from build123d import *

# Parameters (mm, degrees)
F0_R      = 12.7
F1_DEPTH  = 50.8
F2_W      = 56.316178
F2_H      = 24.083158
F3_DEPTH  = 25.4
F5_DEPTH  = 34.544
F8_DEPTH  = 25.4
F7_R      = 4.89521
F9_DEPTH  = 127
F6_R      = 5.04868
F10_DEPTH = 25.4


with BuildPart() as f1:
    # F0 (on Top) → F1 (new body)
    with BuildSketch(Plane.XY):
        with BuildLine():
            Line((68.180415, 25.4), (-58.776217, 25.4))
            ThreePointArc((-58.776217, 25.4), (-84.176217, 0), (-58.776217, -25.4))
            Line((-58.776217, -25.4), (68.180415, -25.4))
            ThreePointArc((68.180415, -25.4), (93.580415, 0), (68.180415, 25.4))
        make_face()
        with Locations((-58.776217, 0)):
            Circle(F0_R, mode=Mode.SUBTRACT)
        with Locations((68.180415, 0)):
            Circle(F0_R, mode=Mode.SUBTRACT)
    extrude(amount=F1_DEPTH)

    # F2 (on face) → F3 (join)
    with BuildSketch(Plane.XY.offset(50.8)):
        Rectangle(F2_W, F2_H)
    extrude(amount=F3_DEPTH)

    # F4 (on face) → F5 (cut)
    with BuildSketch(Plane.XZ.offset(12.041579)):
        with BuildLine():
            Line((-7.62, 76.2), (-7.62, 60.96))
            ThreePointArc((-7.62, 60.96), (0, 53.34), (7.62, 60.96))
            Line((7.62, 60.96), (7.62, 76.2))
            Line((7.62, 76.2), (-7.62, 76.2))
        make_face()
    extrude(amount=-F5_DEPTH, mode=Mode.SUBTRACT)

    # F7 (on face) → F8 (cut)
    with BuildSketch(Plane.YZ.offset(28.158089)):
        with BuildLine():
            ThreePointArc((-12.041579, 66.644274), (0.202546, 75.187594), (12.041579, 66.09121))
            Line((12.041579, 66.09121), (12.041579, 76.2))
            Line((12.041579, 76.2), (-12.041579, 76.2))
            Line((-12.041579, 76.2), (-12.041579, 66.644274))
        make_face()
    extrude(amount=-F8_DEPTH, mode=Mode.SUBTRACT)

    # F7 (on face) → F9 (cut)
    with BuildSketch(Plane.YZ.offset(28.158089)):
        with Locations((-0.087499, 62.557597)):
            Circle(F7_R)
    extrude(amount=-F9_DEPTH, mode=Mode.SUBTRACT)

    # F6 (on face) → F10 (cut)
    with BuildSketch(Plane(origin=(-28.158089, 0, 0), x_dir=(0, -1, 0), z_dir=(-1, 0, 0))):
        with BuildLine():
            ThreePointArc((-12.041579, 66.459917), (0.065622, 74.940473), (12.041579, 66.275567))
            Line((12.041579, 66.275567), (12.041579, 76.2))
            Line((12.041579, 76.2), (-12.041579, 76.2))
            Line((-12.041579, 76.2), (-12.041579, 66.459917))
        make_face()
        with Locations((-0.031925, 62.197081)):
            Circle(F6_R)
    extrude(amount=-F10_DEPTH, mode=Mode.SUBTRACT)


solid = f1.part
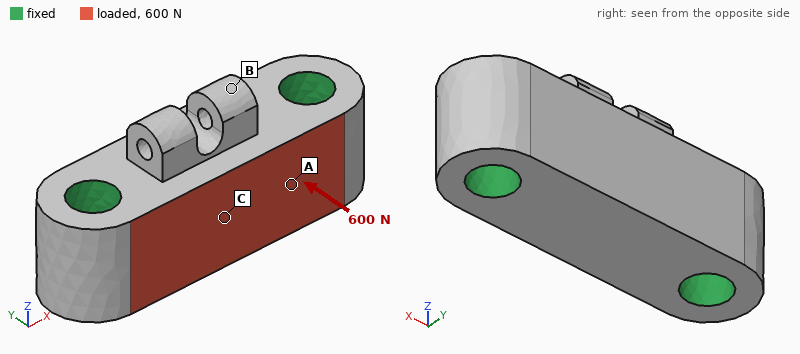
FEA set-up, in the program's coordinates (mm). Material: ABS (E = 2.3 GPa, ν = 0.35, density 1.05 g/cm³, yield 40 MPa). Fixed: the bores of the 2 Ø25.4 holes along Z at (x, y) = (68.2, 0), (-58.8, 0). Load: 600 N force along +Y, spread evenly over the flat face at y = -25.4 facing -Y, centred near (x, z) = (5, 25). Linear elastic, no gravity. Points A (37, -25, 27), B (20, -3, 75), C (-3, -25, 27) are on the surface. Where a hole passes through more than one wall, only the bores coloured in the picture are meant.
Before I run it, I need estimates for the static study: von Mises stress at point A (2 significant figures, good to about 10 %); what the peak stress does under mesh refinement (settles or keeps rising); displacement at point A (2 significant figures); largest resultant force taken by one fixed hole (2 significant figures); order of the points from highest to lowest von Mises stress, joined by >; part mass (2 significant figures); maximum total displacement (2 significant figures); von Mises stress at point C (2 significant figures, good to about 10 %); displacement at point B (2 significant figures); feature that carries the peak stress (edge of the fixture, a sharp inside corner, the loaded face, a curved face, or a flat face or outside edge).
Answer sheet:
0.092 MPa
keeps rising
4.7 µm
300 N
C > A > B
420 g
7.1 µm
0.17 MPa
6.5 µm
edge of the fixture
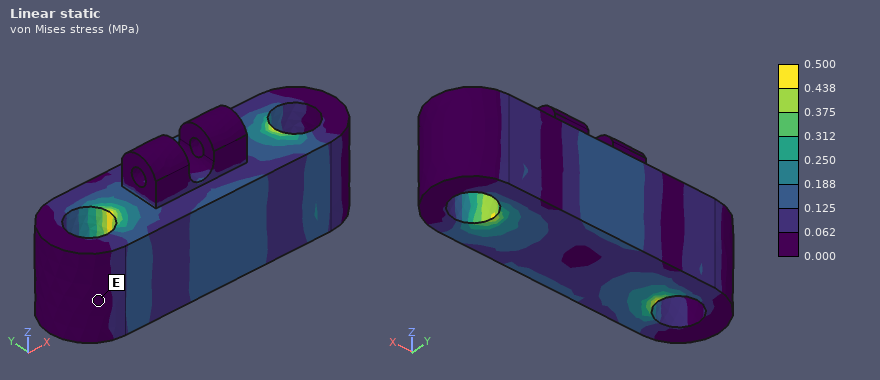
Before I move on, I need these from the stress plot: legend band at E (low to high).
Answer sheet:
0.000 to 0.062 MPa
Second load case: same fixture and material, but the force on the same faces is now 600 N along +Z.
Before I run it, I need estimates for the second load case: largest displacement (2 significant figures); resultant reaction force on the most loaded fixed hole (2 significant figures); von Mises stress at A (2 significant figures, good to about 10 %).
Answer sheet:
15 µm
300 N
0.41 MPa
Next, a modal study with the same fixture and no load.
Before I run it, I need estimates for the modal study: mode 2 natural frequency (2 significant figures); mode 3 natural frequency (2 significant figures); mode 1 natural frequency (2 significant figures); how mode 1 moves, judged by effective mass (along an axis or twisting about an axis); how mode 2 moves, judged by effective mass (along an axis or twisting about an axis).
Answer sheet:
3100 Hz
3300 Hz
2700 Hz
along Y
along Z
